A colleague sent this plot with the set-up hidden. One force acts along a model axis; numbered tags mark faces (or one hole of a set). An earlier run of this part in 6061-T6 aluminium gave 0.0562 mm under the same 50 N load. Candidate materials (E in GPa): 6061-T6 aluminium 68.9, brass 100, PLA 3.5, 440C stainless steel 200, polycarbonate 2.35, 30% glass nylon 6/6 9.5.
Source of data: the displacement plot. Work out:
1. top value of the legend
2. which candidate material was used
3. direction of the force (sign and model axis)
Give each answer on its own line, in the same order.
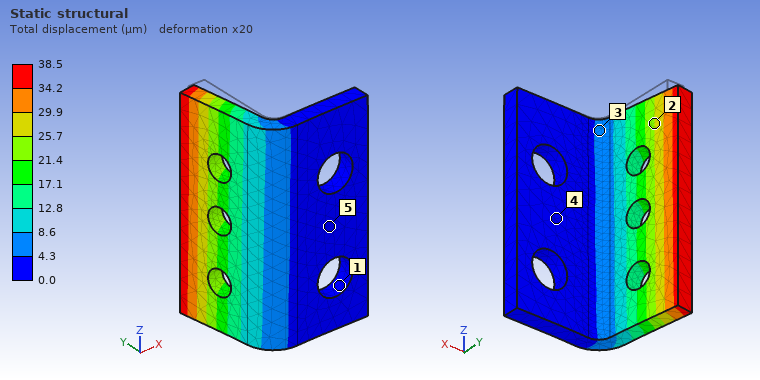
38.5 µm
brass
-X
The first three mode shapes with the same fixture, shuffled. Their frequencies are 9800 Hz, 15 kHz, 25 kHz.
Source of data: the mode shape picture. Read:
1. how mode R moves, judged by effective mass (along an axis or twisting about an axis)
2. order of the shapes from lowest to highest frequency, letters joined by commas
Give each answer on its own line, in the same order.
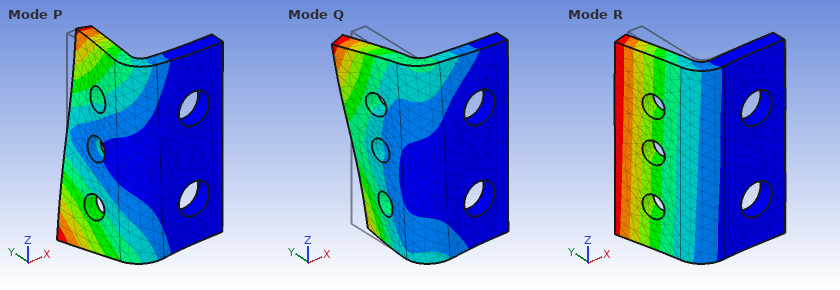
along X
R, P, Q
